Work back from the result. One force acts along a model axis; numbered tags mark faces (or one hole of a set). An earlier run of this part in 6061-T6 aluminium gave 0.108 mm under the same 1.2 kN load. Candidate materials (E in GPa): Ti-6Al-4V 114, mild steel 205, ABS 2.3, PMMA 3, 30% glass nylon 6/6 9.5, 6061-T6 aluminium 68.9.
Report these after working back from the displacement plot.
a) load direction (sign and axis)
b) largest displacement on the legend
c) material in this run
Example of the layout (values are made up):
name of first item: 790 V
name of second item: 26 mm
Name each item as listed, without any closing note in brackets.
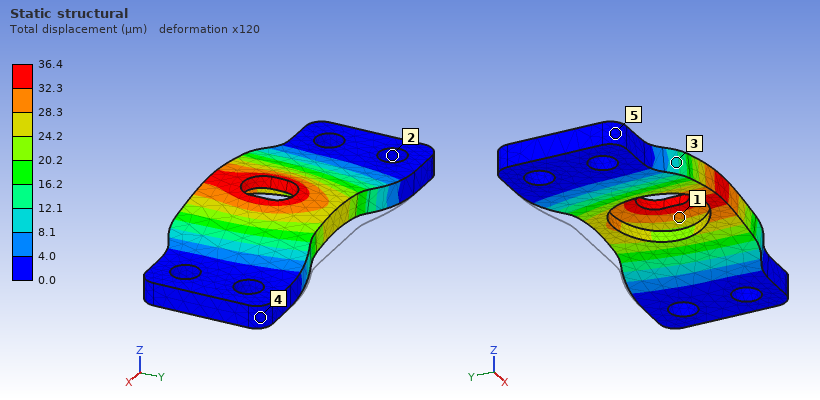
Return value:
load direction: +Z
largest displacement on the legend: 36.4 µm
material in this run: mild steel
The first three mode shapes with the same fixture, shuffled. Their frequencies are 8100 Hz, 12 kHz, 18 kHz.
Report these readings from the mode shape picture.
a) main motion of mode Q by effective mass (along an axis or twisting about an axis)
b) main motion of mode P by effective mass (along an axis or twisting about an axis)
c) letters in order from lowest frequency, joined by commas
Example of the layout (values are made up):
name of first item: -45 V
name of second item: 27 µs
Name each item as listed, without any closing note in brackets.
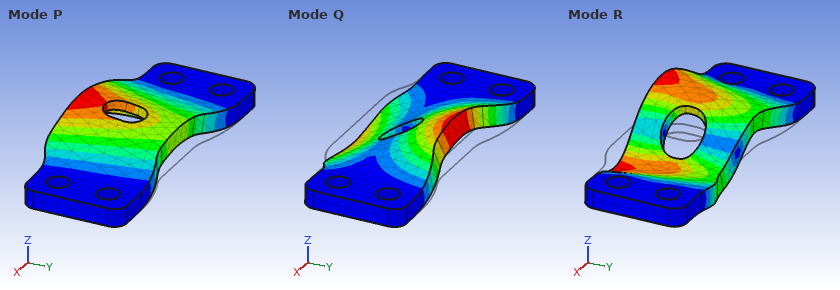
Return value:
main motion of mode Q by effective mass: twisting about X
main motion of mode P by effective mass: along Z
letters in order from lowest frequency, joined by commas: P, Q, R
